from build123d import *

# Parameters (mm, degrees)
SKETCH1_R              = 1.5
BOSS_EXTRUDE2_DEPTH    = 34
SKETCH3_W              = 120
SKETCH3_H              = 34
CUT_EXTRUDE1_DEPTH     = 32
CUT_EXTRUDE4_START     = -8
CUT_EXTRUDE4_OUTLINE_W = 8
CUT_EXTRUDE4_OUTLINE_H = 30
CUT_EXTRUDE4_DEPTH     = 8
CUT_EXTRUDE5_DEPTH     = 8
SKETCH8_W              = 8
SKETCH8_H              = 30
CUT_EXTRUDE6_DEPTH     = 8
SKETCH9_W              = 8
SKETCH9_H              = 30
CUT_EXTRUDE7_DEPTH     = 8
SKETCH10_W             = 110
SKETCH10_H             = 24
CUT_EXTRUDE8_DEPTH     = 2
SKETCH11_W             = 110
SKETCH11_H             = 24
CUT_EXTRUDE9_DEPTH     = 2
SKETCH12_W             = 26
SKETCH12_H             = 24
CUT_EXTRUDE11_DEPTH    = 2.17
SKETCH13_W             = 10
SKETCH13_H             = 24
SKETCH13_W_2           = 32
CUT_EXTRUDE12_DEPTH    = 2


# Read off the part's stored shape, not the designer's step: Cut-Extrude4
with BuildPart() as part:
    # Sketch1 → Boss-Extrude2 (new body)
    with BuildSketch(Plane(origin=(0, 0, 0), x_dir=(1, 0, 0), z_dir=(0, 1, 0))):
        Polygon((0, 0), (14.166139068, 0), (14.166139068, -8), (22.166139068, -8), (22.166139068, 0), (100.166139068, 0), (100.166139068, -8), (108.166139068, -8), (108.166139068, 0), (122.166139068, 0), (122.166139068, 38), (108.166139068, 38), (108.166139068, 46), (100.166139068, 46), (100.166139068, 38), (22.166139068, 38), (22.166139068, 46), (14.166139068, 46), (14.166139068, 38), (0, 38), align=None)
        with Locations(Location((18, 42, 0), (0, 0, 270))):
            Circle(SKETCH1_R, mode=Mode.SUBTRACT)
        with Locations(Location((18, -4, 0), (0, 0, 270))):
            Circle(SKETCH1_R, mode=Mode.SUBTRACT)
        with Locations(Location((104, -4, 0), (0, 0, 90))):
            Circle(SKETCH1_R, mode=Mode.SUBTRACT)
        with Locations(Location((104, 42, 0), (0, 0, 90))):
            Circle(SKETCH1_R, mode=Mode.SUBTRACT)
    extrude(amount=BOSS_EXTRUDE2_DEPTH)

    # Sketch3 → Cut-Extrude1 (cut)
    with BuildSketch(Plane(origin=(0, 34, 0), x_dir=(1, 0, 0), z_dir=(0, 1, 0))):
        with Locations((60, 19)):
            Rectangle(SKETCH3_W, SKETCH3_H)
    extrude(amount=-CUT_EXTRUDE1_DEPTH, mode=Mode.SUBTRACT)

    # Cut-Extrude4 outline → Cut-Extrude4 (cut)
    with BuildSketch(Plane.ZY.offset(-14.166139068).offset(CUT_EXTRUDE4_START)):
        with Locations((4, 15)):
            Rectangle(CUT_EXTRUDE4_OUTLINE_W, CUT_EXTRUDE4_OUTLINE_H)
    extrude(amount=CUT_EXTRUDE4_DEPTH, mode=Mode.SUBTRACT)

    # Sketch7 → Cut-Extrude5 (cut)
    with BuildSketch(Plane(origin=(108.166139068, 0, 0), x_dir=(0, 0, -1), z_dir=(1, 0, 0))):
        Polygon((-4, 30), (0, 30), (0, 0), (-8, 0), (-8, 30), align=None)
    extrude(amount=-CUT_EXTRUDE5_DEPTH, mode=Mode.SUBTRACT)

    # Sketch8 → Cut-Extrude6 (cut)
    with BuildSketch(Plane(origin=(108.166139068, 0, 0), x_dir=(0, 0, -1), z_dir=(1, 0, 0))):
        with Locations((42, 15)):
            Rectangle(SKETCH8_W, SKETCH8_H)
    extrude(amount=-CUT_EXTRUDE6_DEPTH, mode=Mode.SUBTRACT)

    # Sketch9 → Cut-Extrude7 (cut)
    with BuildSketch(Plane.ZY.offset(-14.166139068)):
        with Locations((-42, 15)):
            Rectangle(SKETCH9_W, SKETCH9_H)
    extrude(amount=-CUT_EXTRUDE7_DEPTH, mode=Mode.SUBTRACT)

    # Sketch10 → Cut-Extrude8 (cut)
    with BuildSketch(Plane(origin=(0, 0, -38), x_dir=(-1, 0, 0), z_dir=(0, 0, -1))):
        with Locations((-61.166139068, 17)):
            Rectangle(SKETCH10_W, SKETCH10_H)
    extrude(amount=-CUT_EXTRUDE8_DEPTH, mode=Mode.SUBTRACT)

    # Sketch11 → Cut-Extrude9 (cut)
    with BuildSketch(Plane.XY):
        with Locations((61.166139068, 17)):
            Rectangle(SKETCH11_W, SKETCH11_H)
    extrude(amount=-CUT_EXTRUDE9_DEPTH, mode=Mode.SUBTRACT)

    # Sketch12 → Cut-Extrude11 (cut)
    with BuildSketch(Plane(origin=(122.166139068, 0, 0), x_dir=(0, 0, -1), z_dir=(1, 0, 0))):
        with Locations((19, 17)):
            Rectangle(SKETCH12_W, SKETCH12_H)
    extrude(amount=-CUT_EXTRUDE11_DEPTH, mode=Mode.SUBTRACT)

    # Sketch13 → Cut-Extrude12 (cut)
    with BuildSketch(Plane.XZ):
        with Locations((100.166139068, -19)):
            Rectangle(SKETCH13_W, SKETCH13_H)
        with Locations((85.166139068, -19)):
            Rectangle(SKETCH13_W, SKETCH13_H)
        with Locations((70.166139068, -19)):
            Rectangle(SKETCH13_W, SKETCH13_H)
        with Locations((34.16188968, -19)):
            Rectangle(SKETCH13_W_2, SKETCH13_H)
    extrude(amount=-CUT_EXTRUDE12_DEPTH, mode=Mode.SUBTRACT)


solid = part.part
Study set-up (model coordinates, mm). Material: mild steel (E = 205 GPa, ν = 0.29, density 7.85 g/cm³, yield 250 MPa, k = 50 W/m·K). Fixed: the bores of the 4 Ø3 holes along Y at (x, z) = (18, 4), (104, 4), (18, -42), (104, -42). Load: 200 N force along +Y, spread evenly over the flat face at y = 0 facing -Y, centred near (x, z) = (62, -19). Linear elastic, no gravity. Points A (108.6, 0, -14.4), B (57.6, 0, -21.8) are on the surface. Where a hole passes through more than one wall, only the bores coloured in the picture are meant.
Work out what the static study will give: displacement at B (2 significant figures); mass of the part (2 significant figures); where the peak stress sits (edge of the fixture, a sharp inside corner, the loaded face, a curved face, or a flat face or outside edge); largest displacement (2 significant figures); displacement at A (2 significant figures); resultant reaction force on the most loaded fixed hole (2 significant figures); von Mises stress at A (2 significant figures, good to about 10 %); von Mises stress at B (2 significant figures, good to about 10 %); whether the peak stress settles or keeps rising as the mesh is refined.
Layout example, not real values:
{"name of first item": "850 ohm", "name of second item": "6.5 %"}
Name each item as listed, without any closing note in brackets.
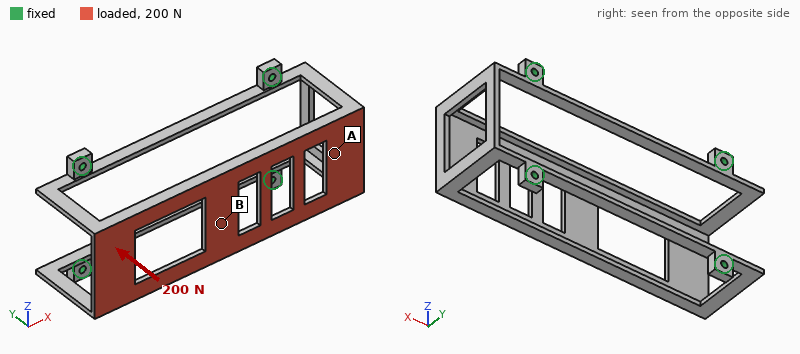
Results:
{"displacement at B": "87 µm", "mass of the part": "100 g", "where the peak stress sits": "a sharp inside corner", "largest displacement": "89 µm", "displacement at A": "28 µm", "resultant reaction force on the most loaded fixed hole": "52 N", "von Mises stress at A": "5.9 MPa", "von Mises stress at B": "14 MPa", "whether the peak stress settles or keeps rising as the mesh is refined": "keeps rising"}
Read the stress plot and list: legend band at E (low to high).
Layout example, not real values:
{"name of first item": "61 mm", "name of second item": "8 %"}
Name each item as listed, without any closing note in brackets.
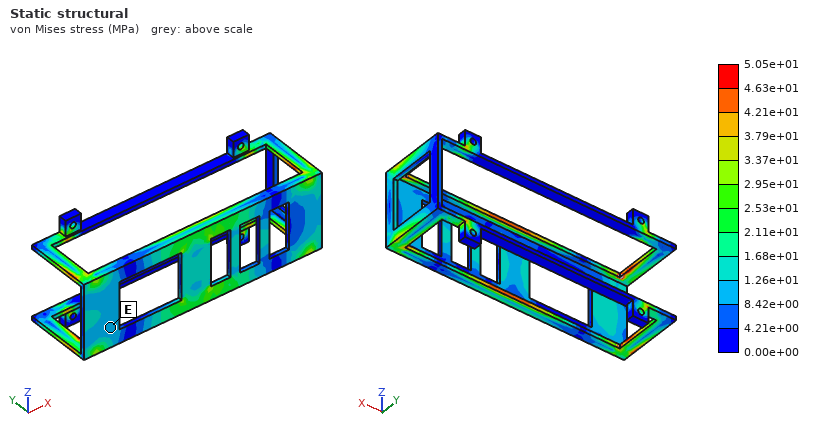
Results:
{"legend band at E": "8.42e+00 to 1.26e+01 MPa"}
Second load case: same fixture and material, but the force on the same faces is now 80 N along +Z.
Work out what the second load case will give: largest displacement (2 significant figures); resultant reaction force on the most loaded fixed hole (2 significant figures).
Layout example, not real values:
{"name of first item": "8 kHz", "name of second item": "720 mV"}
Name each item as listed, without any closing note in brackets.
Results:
{"largest displacement": "0.11 mm", "resultant reaction force on the most loaded fixed hole": "44 N"}
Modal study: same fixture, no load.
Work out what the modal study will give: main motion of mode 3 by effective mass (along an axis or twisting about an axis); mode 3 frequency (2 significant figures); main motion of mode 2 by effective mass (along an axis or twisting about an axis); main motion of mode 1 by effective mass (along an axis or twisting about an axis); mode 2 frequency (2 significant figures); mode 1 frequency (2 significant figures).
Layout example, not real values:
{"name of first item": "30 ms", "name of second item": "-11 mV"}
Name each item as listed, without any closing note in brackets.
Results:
{"main motion of mode 3 by effective mass": "along Y", "mode 3 frequency": "1100 Hz", "main motion of mode 2 by effective mass": "along X", "main motion of mode 1 by effective mass": "along Z", "mode 2 frequency": "920 Hz", "mode 1 frequency": "610 Hz"}
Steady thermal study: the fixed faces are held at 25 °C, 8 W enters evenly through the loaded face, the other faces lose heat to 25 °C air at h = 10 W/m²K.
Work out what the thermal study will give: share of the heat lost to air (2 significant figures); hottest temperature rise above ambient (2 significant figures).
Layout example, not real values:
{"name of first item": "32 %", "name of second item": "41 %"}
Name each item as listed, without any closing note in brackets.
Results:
{"share of the heat lost to air": "61 %", "hottest temperature rise above ambient": "75 K"}
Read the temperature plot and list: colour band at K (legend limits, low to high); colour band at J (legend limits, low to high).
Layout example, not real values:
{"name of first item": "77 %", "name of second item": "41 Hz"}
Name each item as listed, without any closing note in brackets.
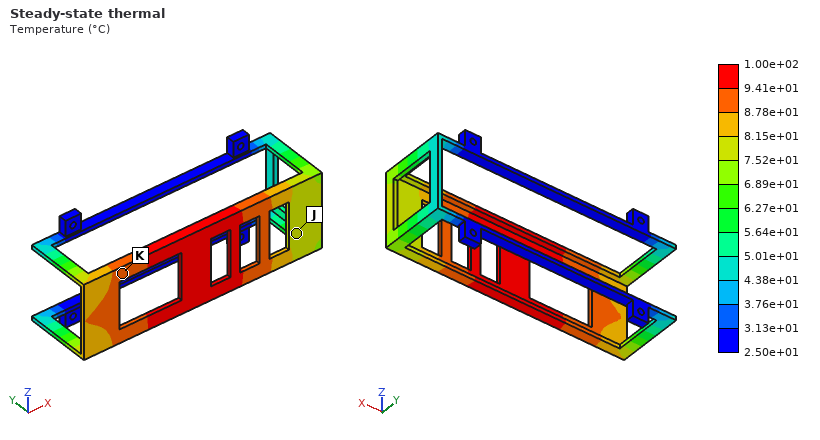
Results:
{"colour band at K": "8.78e+01 to 9.41e+01 °C", "colour band at J": "7.52e+01 to 8.15e+01 °C"}
